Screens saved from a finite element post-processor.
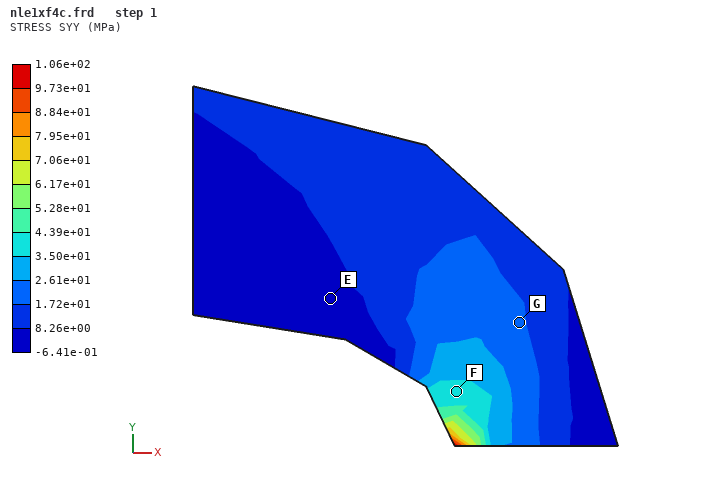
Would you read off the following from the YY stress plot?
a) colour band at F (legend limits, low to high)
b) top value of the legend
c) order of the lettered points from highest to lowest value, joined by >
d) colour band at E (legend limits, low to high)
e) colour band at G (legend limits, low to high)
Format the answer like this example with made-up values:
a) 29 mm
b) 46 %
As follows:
a) 3.50e+01 to 4.39e+01 MPa
b) 1.06e+02 MPa
c) F > G > E
d) -6.41e-01 to 8.26e+00 MPa
e) 1.72e+01 to 2.61e+01 MPa
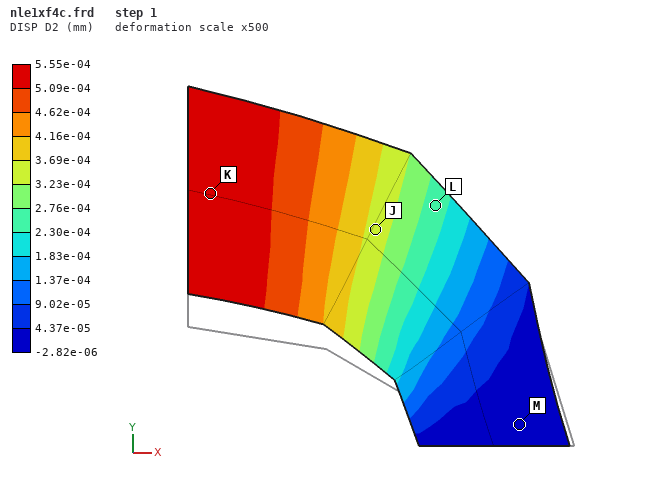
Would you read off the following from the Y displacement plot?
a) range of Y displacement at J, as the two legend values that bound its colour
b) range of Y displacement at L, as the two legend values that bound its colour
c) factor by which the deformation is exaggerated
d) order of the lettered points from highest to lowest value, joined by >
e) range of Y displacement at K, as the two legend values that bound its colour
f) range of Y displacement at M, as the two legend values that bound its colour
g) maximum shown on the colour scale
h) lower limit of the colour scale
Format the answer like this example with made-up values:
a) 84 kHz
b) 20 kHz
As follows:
a) 3.23e-04 to 3.69e-04 mm
b) 2.30e-04 to 2.76e-04 mm
c) 500
d) K > J > L > M
e) 5.09e-04 to 5.55e-04 mm
f) -2.82e-06 to 4.37e-05 mm
g) 5.55e-04 mm
h) -2.82e-06 mm
